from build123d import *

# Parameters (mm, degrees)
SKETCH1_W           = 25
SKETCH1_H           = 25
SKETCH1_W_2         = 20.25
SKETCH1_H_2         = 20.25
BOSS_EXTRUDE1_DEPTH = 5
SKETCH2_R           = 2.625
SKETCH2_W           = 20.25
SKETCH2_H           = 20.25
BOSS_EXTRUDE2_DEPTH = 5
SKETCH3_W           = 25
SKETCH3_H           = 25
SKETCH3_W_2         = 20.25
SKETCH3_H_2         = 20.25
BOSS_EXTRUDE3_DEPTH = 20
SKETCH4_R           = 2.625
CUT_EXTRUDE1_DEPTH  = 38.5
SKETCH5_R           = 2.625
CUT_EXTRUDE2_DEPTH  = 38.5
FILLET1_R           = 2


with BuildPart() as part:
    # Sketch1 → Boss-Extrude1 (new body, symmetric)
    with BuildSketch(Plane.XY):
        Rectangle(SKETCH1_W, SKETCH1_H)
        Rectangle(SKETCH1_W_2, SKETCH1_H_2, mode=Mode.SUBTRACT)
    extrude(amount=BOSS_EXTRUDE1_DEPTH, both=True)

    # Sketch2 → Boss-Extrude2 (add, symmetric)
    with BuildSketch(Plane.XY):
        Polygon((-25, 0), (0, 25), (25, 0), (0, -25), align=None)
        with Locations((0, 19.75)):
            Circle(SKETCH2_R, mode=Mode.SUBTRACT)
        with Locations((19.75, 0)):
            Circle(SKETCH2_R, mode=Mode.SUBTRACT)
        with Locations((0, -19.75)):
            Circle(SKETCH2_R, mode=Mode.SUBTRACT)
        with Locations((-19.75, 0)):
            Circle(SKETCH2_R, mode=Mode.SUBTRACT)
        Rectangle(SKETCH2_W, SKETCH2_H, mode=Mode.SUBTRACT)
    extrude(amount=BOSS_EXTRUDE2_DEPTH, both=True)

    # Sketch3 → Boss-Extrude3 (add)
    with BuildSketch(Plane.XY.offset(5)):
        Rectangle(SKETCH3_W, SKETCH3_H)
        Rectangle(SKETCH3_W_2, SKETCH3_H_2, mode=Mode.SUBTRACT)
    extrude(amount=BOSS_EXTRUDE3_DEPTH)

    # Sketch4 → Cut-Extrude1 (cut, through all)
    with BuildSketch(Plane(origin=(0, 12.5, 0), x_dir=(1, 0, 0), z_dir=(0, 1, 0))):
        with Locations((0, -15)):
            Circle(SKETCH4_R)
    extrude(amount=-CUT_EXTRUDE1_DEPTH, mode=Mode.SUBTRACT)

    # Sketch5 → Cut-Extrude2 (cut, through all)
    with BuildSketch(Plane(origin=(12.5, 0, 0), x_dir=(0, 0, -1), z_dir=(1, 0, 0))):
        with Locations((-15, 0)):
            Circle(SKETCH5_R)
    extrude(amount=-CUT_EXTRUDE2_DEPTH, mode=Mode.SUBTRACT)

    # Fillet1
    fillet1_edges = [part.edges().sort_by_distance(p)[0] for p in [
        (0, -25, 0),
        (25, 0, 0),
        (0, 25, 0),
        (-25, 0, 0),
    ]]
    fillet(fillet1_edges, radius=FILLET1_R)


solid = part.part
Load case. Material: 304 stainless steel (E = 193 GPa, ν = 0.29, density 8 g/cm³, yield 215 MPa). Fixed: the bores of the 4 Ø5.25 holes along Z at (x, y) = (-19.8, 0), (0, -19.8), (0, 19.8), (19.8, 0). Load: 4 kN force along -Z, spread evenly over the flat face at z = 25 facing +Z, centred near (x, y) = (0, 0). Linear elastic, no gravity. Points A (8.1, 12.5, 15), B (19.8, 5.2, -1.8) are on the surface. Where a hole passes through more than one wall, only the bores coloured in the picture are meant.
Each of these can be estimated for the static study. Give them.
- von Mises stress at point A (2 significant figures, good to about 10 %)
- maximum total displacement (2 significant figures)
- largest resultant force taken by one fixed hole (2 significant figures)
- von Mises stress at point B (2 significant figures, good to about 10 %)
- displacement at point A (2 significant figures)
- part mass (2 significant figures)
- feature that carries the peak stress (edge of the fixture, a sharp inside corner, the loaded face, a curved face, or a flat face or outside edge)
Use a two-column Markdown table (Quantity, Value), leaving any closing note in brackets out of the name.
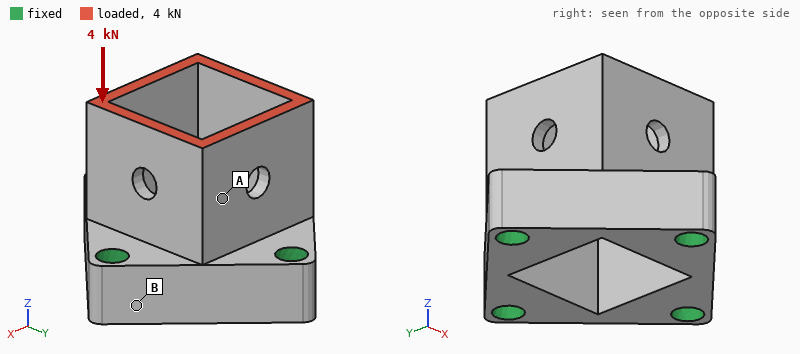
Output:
| Quantity | Value |
|---|---|
| von Mises stress at point A | 18 MPa |
| maximum total displacement | 3.7 µm |
| largest resultant force taken by one fixed hole | 1.0 kN |
| von Mises stress at point B | 7.2 MPa |
| displacement at point A | 2.4 µm |
| part mass | 93 g |
| feature that carries the peak stress | a curved face |
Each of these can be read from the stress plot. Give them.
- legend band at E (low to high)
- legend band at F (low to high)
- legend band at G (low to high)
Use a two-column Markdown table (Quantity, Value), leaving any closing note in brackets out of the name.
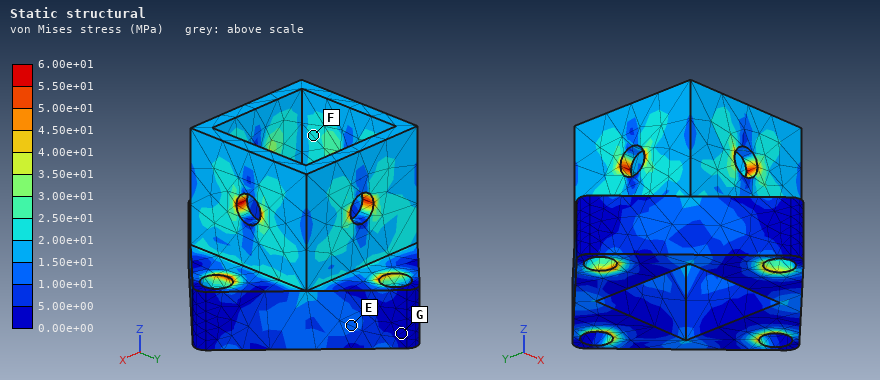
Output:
| Quantity | Value |
|---|---|
| legend band at E | 1.00e+01 to 1.50e+01 MPa |
| legend band at F | 2.00e+01 to 2.50e+01 MPa |
| legend band at G | 0.00e+00 to 5.00e+00 MPa |
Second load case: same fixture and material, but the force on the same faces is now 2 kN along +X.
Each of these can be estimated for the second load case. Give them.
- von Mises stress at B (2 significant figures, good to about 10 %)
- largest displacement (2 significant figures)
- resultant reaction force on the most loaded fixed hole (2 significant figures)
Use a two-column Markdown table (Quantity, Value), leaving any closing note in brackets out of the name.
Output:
| Quantity | Value |
|---|---|
| von Mises stress at B | 15 MPa |
| largest displacement | 33 µm |
| resultant reaction force on the most loaded fixed hole | 1.4 kN |
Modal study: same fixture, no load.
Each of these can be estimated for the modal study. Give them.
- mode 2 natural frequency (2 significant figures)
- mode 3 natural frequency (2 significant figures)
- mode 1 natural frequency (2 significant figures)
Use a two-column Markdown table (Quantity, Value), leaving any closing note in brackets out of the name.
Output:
| Quantity | Value |
|---|---|
| mode 2 natural frequency | 15 kHz |
| mode 3 natural frequency | 15 kHz |
| mode 1 natural frequency | 14 kHz |
